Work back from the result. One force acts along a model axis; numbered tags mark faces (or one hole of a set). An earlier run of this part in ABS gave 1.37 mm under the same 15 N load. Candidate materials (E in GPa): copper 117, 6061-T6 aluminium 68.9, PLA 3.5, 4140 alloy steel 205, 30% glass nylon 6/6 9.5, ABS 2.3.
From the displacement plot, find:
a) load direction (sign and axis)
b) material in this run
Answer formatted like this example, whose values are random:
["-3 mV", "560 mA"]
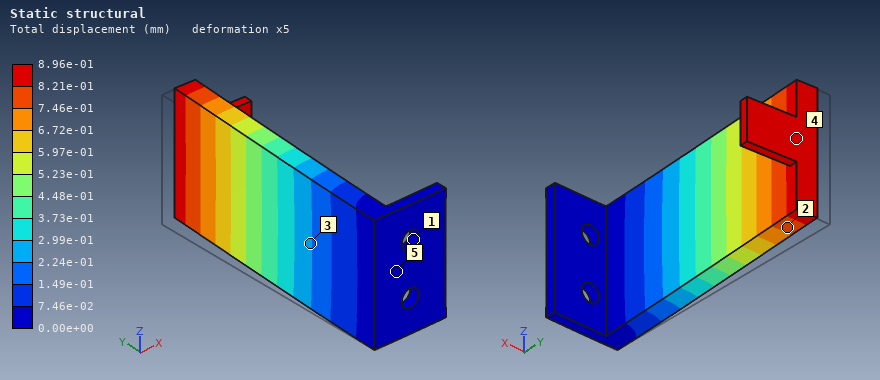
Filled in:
["+X", "PLA"]
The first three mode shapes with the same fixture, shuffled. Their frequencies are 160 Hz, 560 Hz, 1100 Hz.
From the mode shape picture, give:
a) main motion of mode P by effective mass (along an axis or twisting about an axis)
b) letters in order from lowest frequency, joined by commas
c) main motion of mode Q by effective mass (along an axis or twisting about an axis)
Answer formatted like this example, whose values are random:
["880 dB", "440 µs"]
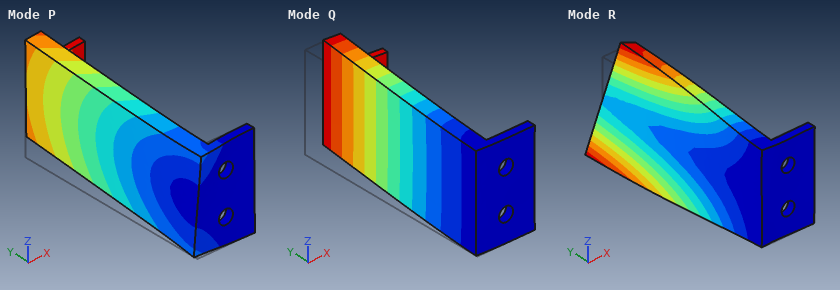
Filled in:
["along Z", "Q, P, R", "along X"]
